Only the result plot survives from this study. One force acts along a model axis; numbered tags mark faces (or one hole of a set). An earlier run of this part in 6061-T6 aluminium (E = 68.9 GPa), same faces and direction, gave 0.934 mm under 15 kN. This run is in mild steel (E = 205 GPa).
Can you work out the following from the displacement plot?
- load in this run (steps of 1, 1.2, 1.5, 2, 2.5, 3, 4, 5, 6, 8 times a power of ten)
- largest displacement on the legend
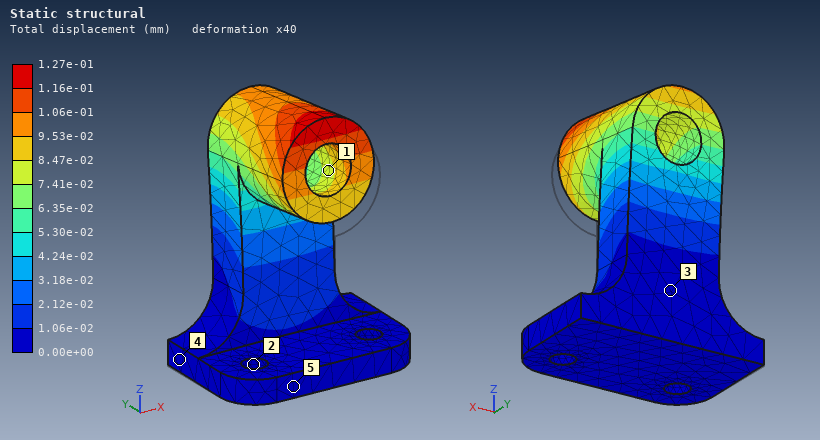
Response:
6 kN
1.27e-01 mm
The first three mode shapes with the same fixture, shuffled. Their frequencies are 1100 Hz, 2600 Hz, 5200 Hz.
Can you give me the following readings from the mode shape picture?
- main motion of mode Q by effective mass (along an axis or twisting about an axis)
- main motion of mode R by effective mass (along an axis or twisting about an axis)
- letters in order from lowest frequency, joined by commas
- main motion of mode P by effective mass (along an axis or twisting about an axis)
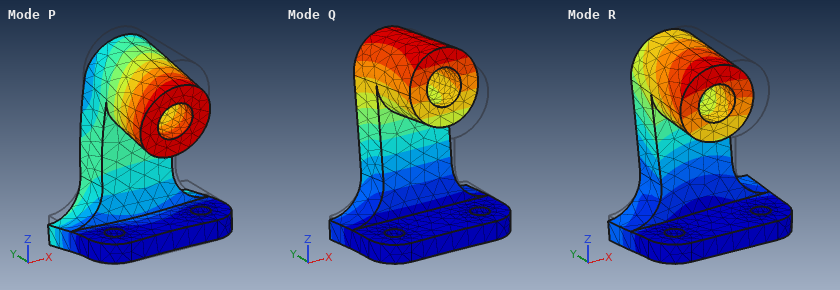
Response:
along Y
along X
Q, R, P
along Z
